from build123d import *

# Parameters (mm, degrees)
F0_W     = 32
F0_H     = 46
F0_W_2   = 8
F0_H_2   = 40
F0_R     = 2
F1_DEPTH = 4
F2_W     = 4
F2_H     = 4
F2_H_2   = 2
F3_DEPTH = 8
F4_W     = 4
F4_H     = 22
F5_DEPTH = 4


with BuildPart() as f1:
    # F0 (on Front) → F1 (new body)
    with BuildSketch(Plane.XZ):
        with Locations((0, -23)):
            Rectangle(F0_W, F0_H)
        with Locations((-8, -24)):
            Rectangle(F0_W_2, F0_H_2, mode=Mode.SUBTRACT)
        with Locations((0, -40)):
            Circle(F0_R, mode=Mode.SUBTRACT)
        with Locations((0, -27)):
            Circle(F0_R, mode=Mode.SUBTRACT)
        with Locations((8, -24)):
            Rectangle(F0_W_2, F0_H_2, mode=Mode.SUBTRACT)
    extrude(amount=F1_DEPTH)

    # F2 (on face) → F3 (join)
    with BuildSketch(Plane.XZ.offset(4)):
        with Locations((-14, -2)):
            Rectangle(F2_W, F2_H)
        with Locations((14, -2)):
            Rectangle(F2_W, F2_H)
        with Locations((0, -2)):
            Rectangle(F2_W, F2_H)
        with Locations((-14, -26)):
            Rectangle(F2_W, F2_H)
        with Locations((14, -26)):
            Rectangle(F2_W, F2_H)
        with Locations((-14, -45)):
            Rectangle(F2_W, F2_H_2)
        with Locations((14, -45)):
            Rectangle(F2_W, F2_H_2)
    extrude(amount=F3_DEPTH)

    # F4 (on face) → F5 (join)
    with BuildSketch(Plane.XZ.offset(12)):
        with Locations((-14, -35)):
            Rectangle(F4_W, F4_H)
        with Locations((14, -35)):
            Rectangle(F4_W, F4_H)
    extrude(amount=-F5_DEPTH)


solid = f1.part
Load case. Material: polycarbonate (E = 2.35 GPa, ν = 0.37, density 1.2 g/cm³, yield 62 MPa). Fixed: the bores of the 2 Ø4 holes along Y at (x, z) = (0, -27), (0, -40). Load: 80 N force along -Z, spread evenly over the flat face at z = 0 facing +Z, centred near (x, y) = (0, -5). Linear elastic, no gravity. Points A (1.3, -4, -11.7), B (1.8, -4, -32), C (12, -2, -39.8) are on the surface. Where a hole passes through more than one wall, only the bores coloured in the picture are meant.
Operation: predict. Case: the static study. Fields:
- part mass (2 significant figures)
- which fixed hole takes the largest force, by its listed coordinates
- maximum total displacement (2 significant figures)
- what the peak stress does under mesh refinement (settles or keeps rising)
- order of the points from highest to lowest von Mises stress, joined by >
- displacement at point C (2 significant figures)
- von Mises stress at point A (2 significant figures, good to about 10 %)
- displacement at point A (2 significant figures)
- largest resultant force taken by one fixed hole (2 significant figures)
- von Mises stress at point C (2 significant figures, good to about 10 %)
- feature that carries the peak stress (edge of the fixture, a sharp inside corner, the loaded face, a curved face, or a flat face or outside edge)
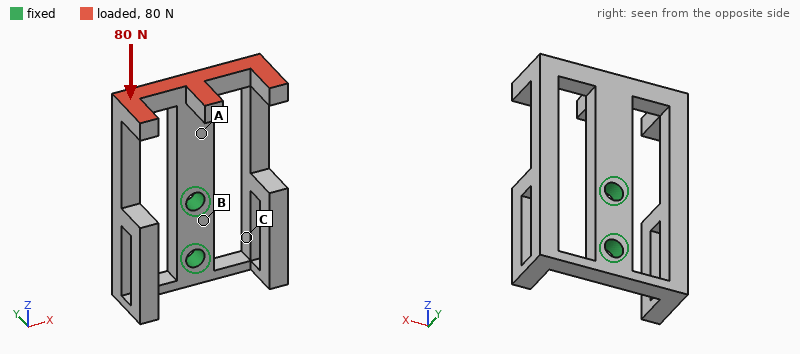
5.4 g
(0, -27)
0.58 mm
keeps rising
A > C > B
0.11 mm
6.9 MPa
0.14 mm
66 N
2.5 MPa
edge of the fixture
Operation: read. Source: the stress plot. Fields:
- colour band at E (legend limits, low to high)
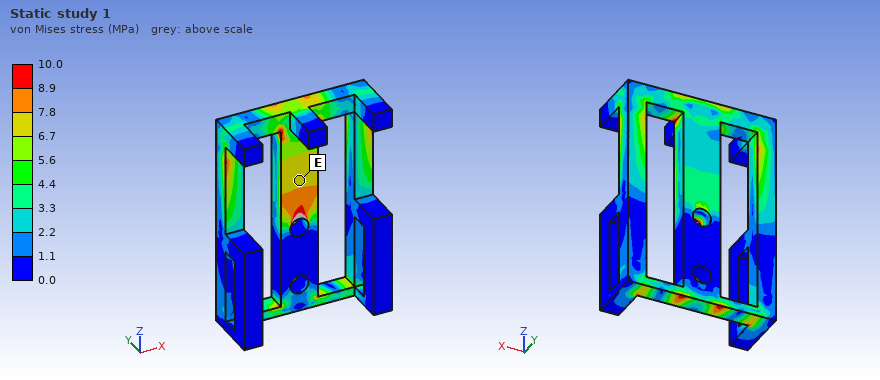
6.7 to 7.8 MPa
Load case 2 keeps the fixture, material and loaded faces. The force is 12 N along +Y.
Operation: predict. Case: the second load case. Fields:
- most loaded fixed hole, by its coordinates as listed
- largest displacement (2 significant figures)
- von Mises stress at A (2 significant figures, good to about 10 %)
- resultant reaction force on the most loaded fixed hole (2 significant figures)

(0, -27)
0.62 mm
4.2 MPa
14 N
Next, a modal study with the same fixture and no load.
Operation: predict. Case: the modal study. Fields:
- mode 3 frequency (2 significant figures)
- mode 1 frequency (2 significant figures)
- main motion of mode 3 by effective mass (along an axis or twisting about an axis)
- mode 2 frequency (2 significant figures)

870 Hz
590 Hz
along X
610 Hz
